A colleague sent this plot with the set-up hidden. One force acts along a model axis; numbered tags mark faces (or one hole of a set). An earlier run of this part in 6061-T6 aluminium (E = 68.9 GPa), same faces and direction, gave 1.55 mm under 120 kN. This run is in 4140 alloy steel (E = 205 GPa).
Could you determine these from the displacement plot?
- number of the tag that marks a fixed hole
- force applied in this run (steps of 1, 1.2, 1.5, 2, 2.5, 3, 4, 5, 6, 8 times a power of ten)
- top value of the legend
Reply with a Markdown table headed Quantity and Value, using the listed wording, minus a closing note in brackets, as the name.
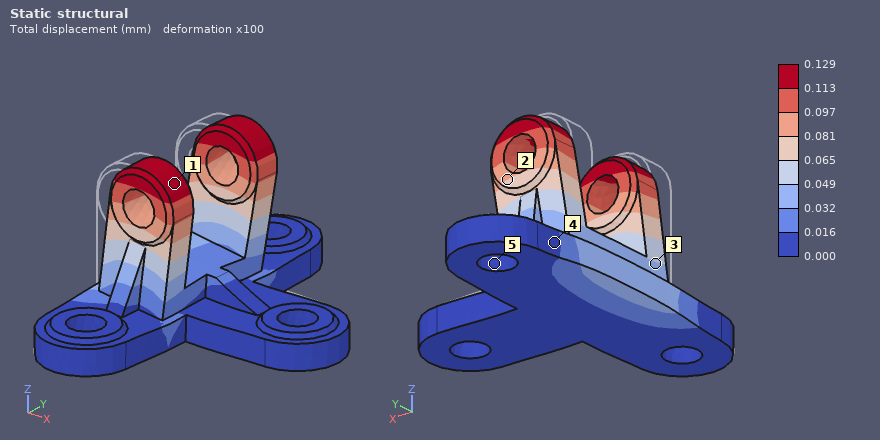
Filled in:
| Quantity | Value |
|---|---|
| number of the tag that marks a fixed hole | 5 |
| force applied in this run | 30 kN |
| top value of the legend | 0.129 mm |
